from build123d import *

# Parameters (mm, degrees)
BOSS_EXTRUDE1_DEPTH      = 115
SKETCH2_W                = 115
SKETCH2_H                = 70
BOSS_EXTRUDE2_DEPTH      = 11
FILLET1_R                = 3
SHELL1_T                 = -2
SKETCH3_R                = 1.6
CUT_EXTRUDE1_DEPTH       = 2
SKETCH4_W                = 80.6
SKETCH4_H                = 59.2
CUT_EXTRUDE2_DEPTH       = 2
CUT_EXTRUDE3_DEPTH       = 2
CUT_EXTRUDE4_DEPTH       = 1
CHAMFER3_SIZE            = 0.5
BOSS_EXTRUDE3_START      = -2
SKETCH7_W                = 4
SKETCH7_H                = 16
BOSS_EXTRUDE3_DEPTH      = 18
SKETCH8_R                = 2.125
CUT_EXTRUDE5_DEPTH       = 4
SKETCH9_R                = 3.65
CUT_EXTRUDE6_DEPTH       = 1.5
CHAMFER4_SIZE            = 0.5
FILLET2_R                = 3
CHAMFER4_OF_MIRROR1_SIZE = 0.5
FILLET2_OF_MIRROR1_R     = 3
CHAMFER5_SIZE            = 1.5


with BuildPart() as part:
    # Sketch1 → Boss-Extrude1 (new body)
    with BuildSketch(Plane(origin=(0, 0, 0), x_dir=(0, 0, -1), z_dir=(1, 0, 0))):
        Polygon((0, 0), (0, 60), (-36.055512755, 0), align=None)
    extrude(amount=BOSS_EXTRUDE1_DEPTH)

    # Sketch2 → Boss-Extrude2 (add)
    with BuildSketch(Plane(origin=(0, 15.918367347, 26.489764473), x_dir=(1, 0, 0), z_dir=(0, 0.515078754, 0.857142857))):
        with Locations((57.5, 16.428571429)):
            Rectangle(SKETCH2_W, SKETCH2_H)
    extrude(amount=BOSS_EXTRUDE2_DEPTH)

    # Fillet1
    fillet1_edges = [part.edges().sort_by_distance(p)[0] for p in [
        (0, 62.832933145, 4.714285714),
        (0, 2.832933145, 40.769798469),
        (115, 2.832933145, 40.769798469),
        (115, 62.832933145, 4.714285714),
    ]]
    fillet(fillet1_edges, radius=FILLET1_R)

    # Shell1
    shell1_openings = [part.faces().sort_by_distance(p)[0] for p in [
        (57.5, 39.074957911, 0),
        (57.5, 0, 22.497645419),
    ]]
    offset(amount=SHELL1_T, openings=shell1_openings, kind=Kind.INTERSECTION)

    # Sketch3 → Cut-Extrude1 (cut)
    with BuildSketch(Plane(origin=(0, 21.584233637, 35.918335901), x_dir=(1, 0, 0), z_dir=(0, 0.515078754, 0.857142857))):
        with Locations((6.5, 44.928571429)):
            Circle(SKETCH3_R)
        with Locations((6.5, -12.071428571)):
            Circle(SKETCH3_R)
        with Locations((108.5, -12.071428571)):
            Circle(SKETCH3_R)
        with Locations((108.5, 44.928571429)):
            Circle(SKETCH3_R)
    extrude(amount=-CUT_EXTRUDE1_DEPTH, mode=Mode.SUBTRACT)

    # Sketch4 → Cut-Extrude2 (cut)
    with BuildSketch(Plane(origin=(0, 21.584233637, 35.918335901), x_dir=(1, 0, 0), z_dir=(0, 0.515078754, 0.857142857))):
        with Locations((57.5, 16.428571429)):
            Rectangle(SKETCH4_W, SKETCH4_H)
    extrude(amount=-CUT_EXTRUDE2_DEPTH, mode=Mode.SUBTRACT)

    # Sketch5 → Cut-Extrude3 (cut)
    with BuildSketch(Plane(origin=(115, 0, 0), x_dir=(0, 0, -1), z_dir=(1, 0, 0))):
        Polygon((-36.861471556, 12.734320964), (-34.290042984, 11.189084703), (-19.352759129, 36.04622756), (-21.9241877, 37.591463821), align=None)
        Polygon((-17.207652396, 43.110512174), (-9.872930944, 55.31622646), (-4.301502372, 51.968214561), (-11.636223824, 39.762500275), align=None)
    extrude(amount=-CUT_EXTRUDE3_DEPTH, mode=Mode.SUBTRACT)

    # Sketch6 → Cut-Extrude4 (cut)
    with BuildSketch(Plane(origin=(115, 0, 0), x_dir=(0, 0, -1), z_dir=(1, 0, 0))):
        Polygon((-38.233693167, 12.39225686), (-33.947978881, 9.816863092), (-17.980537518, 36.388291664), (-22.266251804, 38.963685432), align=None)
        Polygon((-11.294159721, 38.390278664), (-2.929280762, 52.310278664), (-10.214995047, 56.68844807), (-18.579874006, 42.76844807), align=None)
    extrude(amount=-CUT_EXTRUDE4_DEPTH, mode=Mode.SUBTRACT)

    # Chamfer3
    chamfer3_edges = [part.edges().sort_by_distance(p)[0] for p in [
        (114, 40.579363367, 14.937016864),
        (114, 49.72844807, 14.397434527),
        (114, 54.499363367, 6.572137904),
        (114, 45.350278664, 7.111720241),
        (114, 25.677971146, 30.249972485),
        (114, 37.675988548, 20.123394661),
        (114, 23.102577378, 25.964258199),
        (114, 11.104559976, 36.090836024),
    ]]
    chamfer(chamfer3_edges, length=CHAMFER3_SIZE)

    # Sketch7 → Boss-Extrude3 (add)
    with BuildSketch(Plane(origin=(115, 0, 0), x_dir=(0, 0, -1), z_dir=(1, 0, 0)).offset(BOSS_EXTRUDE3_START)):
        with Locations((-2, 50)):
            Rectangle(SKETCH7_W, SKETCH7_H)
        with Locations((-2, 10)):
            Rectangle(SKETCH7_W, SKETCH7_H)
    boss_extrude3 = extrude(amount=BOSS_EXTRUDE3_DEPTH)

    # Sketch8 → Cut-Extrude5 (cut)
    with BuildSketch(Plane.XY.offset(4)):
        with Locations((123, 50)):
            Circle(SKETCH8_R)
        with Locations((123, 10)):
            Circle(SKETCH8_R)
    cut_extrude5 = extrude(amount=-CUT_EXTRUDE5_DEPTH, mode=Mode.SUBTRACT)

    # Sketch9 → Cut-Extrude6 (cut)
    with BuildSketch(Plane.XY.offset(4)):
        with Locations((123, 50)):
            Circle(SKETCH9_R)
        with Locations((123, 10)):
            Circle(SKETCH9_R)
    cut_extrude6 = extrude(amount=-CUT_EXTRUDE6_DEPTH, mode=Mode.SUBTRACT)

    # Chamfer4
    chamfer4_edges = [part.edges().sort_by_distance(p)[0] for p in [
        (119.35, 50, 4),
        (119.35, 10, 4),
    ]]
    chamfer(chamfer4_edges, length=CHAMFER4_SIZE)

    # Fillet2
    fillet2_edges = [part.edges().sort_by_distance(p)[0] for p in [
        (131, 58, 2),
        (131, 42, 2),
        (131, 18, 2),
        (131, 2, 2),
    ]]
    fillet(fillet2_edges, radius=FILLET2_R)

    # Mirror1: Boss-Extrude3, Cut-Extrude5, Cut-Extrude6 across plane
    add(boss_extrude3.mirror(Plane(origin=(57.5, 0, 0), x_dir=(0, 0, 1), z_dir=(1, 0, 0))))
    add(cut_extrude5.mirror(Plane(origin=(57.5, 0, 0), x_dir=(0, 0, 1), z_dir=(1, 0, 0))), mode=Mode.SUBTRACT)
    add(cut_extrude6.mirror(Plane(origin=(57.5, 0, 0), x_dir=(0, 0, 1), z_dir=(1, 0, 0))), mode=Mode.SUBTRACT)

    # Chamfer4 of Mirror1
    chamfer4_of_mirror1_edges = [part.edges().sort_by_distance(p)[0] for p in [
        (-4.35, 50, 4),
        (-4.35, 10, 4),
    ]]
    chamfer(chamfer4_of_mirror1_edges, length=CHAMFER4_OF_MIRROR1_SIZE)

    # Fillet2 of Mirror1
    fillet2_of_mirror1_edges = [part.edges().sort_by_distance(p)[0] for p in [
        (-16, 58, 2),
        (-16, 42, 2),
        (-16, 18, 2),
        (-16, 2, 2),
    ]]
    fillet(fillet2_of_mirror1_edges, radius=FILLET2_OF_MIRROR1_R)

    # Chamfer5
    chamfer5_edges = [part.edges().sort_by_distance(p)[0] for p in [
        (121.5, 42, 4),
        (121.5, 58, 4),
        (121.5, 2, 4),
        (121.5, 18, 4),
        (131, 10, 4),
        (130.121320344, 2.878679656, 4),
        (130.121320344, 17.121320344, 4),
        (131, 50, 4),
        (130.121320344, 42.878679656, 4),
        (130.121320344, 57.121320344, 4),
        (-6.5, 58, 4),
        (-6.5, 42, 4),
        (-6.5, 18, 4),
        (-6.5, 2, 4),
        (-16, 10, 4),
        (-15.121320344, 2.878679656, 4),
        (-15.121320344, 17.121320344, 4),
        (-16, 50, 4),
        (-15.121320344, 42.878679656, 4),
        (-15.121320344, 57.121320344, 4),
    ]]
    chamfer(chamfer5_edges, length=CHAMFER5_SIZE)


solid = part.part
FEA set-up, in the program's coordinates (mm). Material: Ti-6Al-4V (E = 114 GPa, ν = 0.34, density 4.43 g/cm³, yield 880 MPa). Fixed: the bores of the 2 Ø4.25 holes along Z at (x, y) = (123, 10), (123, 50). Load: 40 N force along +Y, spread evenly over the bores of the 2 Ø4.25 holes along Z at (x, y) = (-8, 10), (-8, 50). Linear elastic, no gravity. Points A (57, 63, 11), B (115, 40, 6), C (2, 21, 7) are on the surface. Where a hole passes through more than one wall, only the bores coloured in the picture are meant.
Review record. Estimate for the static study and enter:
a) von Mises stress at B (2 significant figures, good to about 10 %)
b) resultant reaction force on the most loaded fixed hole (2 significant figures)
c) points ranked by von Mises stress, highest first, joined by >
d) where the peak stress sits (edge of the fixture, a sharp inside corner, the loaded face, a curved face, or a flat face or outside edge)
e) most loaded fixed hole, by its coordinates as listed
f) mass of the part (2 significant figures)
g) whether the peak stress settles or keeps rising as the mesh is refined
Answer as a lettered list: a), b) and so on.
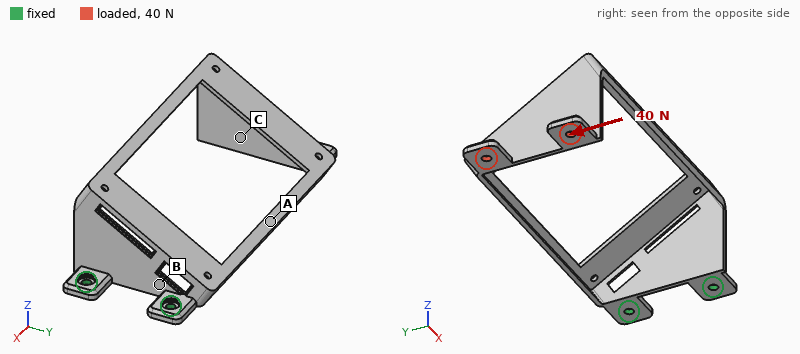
a) 32 MPa
b) 100 N
c) B > A > C
d) a sharp inside corner
e) (123, 10)
f) 92 g
g) keeps rising
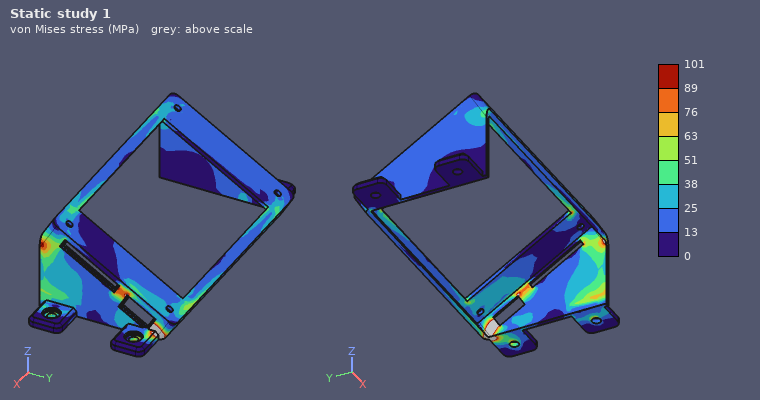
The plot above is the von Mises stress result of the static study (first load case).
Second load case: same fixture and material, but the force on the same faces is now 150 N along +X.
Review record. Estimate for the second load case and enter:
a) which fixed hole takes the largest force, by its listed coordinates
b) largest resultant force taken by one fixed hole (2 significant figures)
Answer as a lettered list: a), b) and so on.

a) (123, 50)
b) 82 N
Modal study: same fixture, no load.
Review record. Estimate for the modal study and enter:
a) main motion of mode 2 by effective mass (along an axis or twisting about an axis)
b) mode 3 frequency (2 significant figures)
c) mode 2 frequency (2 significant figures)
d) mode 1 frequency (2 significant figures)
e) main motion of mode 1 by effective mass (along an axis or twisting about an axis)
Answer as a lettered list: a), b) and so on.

a) along Y
b) 360 Hz
c) 150 Hz
d) 100 Hz
e) along Z
